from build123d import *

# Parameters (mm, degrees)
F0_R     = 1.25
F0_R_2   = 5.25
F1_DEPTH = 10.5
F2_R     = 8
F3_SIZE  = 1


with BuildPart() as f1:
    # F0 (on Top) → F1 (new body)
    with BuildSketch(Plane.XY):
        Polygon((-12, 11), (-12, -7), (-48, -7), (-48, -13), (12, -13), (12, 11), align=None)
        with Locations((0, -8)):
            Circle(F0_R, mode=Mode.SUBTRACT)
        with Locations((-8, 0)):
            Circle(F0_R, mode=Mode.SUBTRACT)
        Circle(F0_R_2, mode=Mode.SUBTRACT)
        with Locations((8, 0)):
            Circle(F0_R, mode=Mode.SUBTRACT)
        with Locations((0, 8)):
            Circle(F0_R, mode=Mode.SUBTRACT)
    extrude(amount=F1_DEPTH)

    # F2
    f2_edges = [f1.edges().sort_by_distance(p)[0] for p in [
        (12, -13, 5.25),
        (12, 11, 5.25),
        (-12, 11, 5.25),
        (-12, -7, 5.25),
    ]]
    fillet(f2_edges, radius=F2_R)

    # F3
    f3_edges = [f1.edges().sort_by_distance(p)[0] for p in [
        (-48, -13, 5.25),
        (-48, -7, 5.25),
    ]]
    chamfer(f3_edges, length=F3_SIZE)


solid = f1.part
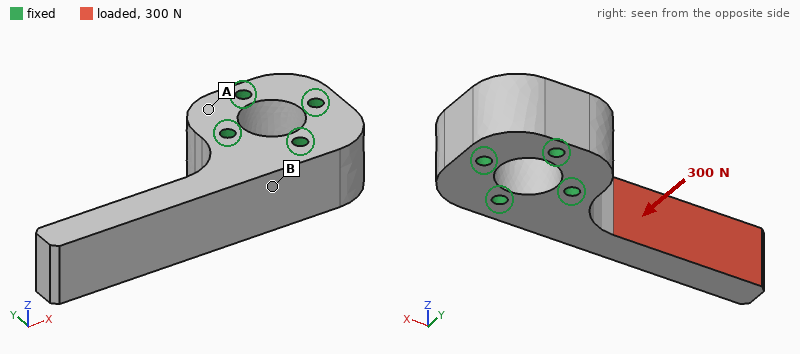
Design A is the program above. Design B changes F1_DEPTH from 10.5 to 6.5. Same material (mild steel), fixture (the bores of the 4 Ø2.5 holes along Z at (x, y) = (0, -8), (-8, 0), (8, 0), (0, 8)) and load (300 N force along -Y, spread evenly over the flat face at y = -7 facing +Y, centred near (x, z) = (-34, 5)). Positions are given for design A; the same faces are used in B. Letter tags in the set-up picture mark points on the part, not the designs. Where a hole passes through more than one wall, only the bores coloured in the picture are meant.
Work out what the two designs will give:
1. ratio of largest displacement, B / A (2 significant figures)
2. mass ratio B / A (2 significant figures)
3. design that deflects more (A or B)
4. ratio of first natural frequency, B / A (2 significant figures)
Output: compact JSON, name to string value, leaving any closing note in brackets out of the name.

{"ratio of largest displacement, B / A": "1.6", "mass ratio B / A": "0.62", "design that deflects more": "B", "ratio of first natural frequency, B / A": "0.83"}
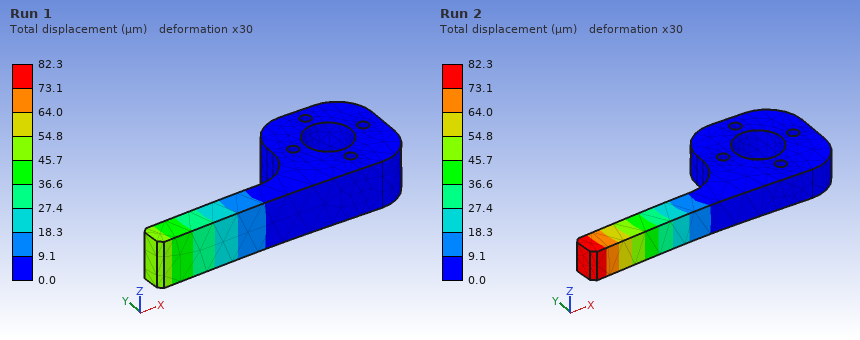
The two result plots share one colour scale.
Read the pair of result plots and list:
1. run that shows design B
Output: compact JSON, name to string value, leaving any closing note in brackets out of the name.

{"run that shows design B": "Run 2"}
